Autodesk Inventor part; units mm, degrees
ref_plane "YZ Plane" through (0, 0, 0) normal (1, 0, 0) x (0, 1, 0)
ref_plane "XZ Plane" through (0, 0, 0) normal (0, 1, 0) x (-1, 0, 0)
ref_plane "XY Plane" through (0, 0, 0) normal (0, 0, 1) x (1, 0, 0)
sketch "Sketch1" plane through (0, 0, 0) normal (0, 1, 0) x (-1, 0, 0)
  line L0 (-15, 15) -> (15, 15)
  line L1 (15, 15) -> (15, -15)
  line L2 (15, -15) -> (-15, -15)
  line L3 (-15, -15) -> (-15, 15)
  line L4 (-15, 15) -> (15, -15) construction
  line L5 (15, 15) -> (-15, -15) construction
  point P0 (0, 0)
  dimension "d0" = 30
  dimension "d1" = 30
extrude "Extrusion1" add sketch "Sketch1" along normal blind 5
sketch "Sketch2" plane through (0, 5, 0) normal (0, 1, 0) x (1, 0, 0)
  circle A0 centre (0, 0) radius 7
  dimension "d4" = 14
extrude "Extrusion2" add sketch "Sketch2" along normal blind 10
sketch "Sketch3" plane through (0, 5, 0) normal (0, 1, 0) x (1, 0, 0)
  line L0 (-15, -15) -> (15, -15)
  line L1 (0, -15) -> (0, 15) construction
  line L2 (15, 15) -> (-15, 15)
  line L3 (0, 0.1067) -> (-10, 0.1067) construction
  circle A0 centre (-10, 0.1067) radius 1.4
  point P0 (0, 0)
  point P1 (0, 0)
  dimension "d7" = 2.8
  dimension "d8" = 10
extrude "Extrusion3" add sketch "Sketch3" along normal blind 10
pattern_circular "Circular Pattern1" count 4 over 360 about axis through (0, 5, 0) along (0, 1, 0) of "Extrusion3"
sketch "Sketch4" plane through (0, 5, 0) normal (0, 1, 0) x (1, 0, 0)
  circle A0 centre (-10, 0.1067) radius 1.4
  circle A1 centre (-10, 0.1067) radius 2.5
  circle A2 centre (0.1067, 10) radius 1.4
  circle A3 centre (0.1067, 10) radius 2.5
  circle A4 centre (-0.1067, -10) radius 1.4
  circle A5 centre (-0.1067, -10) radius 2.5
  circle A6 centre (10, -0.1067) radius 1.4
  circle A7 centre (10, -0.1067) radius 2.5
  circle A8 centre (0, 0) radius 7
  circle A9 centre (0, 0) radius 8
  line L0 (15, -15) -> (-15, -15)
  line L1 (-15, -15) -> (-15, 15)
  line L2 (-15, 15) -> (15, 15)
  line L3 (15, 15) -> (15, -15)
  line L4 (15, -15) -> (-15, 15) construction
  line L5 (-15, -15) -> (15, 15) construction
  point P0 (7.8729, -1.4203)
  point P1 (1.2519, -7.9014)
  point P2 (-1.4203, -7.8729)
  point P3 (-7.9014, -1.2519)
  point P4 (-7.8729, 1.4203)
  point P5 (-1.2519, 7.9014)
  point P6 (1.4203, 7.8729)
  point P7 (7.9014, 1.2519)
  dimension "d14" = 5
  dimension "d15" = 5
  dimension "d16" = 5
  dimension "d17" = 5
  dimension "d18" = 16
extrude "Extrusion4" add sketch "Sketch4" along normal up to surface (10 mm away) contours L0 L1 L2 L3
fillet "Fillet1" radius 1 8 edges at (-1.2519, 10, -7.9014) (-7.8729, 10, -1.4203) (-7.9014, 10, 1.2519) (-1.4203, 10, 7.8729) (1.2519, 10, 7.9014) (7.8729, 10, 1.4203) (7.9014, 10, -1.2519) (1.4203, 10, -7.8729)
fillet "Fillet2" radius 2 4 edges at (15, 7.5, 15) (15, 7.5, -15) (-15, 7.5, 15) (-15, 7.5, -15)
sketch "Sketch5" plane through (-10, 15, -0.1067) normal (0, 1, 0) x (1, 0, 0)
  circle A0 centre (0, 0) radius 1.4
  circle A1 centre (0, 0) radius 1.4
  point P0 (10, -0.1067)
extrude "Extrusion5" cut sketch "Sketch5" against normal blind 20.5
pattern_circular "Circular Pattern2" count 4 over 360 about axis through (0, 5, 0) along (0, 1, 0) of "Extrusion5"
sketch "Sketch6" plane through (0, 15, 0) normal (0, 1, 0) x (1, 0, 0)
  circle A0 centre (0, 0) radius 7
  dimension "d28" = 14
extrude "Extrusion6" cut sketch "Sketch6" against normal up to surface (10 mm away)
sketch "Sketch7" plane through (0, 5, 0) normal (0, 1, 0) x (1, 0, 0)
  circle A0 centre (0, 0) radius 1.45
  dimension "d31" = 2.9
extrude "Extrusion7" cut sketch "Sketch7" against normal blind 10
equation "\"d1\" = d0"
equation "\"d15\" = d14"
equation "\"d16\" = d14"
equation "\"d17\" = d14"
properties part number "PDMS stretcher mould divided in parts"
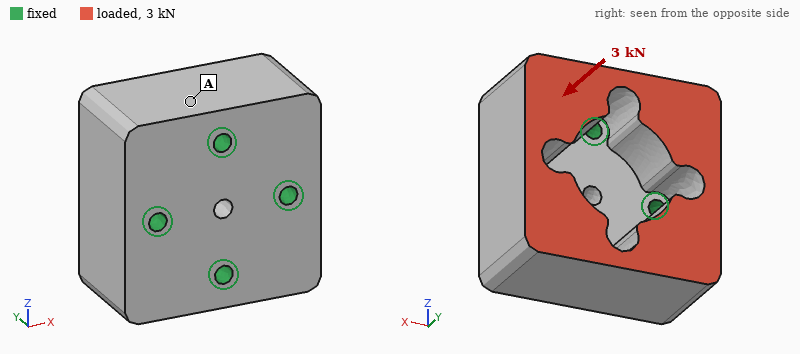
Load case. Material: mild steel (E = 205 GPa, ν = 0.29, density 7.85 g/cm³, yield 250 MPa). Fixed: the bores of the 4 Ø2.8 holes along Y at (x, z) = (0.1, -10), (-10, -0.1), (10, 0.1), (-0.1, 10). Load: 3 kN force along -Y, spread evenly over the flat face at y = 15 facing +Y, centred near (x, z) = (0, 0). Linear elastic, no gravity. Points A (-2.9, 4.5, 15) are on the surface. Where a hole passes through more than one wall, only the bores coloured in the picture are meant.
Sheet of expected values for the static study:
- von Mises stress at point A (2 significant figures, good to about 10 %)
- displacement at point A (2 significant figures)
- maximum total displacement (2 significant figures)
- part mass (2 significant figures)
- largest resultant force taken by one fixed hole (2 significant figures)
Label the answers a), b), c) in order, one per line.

a) 7.1 MPa
b) 0.67 µm
c) 1.6 µm
d) 82 g
e) 750 N
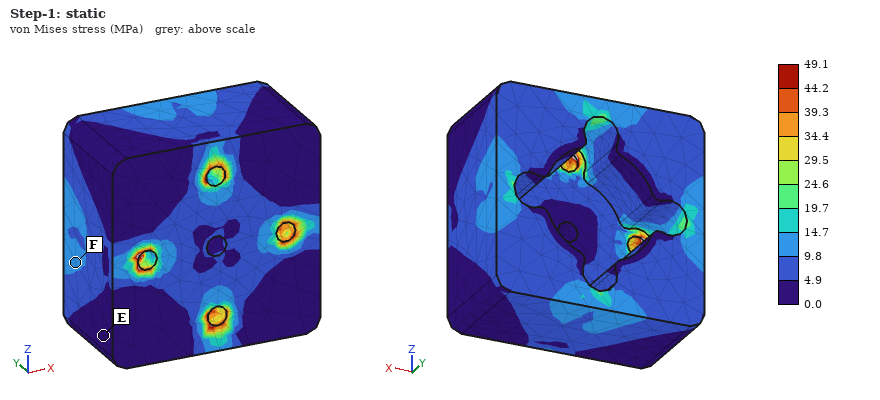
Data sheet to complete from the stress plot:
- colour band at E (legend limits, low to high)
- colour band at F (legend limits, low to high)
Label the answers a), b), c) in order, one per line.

a) 0.0 to 4.9 MPa
b) 9.8 to 14.7 MPa
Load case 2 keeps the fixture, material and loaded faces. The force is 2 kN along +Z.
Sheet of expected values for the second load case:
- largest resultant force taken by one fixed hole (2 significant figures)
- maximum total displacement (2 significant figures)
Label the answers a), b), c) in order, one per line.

a) 970 N
b) 4.4 µm
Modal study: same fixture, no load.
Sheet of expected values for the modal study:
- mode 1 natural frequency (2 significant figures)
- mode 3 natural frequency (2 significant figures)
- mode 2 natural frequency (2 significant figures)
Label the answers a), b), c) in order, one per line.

a) 21 kHz
b) 21 kHz
c) 21 kHz
